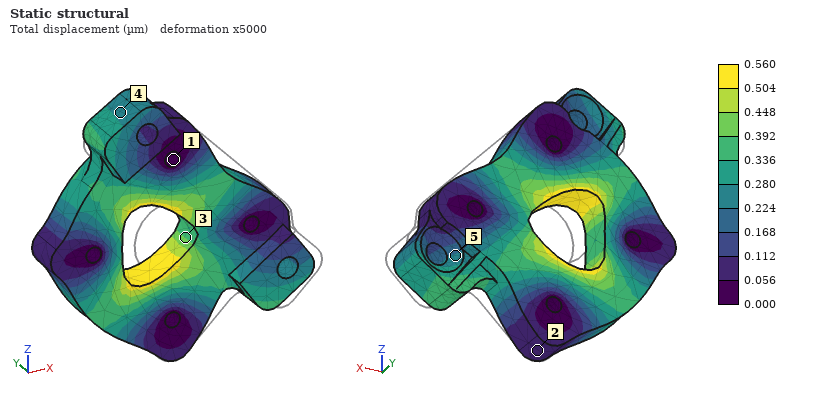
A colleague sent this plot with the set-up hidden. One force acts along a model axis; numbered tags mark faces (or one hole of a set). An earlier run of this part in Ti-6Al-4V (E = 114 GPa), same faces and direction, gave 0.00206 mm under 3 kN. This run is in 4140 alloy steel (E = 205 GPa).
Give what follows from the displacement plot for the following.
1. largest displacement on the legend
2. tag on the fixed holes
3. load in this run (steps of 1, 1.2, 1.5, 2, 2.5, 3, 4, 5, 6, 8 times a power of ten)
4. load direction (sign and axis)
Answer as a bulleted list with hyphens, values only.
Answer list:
- 0.560 µm
- 1
- 1.5 kN
- -X
